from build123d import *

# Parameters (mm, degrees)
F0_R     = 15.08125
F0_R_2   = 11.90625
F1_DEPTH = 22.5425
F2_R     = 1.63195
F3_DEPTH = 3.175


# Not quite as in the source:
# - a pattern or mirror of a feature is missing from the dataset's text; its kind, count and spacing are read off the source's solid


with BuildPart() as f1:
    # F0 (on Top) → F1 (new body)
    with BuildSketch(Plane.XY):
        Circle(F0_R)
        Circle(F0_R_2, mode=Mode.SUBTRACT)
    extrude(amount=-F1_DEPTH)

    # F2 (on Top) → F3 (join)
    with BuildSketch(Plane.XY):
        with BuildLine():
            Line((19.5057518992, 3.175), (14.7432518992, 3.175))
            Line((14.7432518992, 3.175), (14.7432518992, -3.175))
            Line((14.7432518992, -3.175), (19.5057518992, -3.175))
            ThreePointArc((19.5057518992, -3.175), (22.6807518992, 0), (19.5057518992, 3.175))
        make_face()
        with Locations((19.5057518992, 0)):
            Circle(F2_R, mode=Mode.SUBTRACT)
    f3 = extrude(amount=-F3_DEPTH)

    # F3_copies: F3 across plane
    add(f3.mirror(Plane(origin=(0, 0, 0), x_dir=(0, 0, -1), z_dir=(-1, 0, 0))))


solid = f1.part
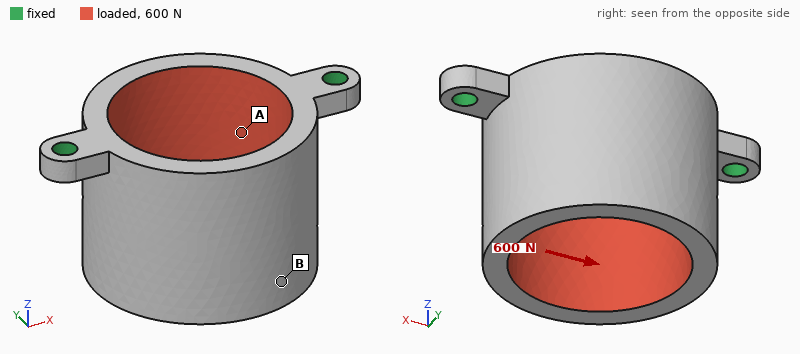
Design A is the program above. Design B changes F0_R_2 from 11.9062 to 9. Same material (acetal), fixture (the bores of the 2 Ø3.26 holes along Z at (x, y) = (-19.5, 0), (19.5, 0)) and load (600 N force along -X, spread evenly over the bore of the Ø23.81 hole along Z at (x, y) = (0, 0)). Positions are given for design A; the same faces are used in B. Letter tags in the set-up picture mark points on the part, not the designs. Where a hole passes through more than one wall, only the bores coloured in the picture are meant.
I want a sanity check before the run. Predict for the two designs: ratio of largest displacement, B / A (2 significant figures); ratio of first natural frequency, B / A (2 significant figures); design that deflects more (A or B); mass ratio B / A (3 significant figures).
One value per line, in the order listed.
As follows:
0.70
0.80
A
1.68
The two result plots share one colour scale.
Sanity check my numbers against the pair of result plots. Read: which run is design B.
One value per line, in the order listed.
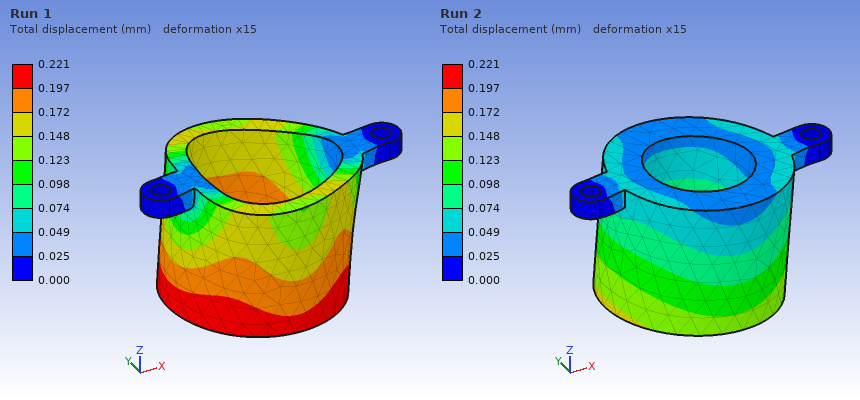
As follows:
Run 2
